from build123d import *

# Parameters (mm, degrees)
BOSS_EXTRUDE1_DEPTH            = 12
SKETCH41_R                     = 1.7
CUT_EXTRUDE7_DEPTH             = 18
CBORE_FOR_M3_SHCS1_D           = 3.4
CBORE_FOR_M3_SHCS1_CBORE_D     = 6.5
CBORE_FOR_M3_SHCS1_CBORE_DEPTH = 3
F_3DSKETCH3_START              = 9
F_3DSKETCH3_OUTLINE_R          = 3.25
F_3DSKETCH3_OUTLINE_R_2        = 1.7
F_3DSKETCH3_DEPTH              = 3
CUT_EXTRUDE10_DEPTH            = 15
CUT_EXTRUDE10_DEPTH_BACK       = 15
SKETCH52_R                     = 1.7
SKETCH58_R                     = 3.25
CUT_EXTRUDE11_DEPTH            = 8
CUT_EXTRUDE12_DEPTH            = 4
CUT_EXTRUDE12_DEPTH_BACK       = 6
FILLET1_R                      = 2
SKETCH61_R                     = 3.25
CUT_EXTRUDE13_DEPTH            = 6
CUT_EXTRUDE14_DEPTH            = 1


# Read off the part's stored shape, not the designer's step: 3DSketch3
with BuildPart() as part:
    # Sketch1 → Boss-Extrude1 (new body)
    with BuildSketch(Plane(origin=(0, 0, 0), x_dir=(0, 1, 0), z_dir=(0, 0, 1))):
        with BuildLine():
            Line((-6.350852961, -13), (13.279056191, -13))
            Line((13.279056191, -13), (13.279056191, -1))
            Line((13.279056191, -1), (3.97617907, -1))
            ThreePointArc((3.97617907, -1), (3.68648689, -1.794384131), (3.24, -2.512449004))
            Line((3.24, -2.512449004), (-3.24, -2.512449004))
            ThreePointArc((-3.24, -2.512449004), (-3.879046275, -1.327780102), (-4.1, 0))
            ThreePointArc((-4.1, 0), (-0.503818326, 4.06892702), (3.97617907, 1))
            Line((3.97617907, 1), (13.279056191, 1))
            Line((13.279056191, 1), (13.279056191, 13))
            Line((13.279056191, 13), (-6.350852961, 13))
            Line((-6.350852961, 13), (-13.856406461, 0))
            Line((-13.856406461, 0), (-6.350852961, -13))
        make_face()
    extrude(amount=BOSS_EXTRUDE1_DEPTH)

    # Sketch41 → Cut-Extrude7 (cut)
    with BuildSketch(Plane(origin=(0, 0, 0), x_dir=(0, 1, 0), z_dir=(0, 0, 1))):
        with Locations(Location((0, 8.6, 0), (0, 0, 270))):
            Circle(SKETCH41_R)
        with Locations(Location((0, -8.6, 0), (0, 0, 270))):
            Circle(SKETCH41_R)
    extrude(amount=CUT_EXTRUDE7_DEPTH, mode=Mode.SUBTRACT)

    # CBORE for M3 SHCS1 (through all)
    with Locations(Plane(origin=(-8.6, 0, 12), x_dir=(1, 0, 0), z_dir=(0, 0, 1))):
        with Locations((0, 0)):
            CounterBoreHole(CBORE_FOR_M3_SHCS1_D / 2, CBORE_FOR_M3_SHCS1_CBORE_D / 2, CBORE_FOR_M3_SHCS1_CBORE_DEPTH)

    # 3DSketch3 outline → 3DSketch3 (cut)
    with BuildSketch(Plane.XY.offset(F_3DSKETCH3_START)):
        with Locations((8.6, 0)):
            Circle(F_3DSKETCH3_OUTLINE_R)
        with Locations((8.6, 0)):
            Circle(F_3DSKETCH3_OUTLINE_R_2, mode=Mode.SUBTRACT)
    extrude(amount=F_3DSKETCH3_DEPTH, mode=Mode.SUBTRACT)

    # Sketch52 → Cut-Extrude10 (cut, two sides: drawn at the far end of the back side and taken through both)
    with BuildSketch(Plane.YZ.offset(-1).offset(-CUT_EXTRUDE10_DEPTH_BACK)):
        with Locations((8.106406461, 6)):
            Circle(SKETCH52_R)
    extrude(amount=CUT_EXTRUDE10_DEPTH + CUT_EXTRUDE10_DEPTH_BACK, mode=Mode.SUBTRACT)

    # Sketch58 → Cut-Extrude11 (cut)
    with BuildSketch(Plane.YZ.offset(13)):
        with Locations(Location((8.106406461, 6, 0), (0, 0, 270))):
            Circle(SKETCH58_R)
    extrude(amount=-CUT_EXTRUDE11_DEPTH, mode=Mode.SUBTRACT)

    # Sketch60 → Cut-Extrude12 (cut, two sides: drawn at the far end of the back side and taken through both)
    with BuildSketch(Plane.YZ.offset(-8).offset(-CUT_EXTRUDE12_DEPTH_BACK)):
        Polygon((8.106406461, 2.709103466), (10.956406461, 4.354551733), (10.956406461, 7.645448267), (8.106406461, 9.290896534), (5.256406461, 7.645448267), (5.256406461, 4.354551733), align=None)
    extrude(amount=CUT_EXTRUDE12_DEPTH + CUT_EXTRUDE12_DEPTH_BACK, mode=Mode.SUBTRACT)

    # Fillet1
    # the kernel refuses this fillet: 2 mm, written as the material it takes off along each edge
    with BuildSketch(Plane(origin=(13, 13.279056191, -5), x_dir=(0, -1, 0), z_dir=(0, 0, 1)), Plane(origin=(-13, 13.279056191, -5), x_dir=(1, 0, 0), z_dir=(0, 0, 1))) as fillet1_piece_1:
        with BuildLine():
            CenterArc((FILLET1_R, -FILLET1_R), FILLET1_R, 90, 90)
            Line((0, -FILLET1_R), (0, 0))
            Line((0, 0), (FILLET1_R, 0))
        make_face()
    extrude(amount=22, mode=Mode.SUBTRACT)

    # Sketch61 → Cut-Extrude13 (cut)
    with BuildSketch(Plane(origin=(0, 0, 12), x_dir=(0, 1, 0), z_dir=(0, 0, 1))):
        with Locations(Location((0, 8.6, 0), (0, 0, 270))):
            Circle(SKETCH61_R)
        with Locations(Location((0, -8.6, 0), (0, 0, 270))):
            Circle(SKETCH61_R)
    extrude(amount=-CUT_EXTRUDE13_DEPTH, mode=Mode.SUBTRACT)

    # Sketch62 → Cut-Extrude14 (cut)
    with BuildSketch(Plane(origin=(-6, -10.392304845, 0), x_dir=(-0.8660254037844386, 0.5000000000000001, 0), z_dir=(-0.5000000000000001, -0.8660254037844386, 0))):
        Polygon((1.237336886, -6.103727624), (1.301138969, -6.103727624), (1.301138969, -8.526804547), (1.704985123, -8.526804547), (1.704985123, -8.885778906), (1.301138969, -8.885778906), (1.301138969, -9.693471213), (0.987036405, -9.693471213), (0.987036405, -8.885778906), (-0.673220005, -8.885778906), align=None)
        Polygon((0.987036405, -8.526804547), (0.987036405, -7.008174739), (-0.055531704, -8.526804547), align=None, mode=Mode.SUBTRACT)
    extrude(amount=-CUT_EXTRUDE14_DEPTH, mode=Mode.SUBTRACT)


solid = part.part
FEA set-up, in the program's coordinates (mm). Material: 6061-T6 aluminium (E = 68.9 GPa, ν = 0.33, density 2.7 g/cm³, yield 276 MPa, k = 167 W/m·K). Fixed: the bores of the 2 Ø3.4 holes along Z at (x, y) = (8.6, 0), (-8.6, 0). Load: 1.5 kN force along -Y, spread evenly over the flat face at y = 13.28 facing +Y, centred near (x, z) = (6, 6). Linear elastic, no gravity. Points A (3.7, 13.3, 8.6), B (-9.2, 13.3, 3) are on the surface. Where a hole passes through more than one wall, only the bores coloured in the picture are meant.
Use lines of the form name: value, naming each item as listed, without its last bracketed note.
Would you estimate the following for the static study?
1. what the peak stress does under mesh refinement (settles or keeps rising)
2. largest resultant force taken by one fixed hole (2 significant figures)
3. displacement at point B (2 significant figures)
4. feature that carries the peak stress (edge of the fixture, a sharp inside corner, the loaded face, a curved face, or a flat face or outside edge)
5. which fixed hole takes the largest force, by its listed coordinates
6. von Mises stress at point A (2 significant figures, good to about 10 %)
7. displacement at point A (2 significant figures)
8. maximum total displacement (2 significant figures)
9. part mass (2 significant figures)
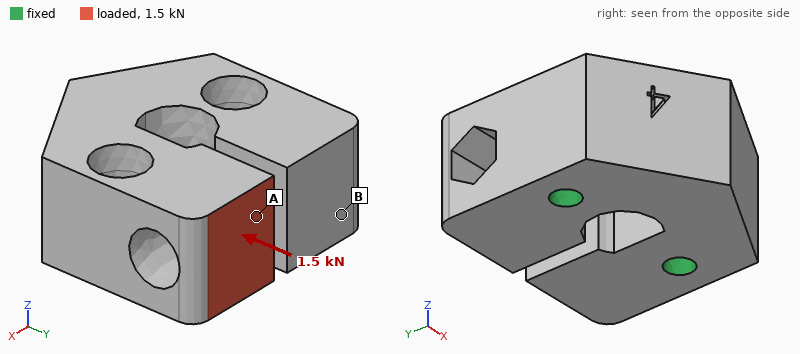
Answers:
what the peak stress does under mesh refinement: keeps rising
largest resultant force taken by one fixed hole: 1.3 kN
displacement at point B: 2.4 µm
feature that carries the peak stress: edge of the fixture
which fixed hole takes the largest force, by its listed coordinates: (8.6, 0)
von Mises stress at point A: 13 MPa
displacement at point A: 13 µm
maximum total displacement: 15 µm
part mass: 15 g
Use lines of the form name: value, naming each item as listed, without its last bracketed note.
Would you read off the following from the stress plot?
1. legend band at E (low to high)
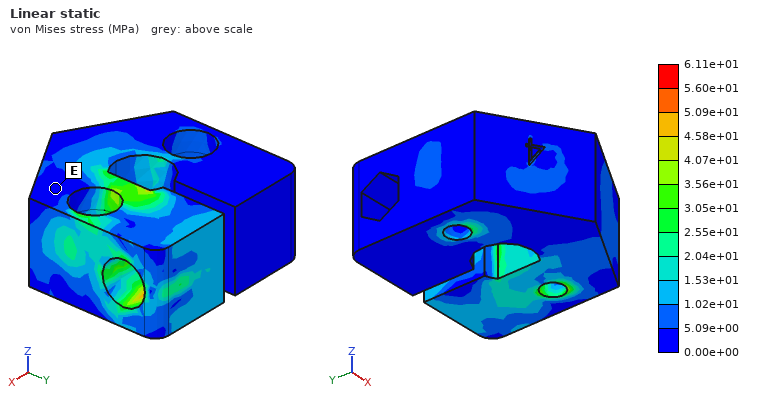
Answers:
legend band at E: 0.00e+00 to 5.09e+00 MPa
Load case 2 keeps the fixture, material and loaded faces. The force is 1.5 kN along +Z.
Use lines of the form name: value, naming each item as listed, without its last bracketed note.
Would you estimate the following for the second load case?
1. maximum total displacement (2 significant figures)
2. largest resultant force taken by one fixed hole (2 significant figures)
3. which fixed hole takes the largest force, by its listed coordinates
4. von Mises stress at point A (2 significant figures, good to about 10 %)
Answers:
maximum total displacement: 68 µm
largest resultant force taken by one fixed hole: 1.6 kN
which fixed hole takes the largest force, by its listed coordinates: (8.6, 0)
von Mises stress at point A: 41 MPa
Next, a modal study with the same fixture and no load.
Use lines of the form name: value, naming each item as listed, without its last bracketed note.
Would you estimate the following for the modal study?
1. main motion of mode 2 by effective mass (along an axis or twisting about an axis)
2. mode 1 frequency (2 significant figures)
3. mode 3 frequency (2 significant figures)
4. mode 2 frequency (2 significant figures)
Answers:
main motion of mode 2 by effective mass: along X
mode 1 frequency: 17 kHz
mode 3 frequency: 21 kHz
mode 2 frequency: 19 kHz
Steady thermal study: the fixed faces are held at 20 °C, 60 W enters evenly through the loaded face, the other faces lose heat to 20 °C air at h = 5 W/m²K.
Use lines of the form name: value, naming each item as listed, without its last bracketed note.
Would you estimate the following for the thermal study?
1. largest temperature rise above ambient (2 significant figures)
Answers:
largest temperature rise above ambient: 60 K
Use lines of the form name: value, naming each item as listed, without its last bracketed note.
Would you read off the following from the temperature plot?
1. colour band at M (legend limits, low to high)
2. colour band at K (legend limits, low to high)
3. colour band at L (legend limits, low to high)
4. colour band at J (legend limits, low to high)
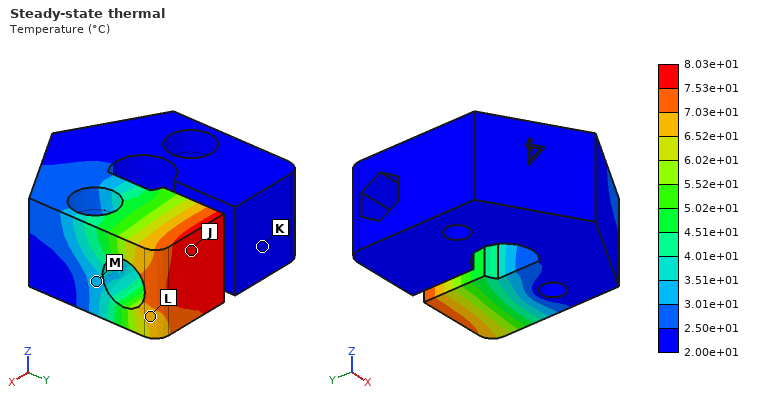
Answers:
colour band at M: 3.01e+01 to 3.51e+01 °C
colour band at K: 2.00e+01 to 2.50e+01 °C
colour band at L: 6.52e+01 to 7.03e+01 °C
colour band at J: 7.53e+01 to 8.03e+01 °C
